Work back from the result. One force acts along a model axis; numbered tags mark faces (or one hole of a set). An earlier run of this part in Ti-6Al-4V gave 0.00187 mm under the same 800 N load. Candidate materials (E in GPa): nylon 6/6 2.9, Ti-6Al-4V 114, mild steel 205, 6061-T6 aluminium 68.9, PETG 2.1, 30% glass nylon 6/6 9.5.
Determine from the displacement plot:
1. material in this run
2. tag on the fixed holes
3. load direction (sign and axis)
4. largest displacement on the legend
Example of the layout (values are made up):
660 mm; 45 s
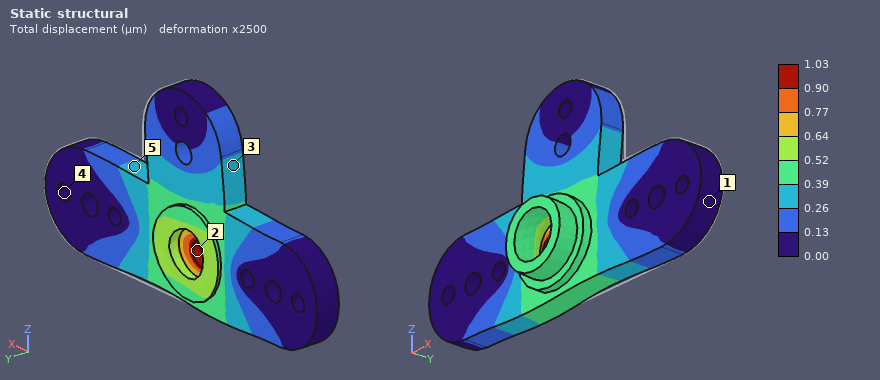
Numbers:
mild steel; 4; -X; 1.03 µm
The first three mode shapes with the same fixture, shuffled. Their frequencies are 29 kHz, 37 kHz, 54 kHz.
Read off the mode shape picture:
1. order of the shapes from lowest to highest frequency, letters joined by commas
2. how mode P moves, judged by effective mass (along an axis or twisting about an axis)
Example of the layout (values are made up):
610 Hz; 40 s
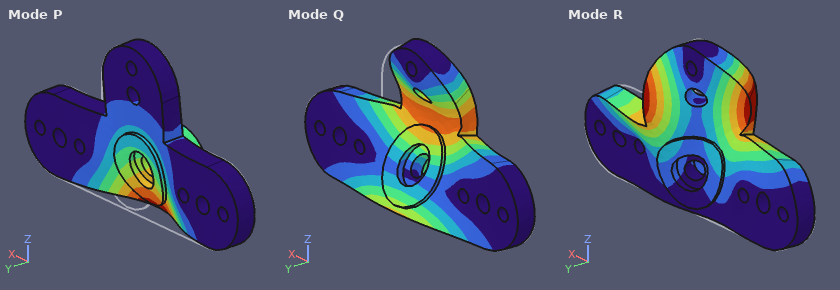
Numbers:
P, Q, R; along Y
